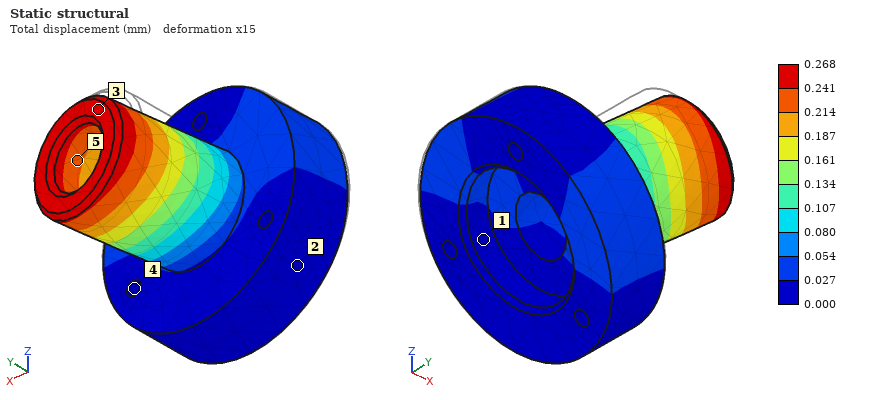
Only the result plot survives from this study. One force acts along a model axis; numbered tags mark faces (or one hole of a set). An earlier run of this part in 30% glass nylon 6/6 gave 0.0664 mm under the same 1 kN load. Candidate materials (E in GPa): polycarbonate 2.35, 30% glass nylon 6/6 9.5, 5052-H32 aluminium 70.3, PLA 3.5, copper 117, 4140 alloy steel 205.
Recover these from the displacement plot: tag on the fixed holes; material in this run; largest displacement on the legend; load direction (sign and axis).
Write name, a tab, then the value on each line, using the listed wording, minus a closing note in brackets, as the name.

tag on the fixed holes	4
material in this run	polycarbonate
largest displacement on the legend	0.268 mm
load direction	+X
